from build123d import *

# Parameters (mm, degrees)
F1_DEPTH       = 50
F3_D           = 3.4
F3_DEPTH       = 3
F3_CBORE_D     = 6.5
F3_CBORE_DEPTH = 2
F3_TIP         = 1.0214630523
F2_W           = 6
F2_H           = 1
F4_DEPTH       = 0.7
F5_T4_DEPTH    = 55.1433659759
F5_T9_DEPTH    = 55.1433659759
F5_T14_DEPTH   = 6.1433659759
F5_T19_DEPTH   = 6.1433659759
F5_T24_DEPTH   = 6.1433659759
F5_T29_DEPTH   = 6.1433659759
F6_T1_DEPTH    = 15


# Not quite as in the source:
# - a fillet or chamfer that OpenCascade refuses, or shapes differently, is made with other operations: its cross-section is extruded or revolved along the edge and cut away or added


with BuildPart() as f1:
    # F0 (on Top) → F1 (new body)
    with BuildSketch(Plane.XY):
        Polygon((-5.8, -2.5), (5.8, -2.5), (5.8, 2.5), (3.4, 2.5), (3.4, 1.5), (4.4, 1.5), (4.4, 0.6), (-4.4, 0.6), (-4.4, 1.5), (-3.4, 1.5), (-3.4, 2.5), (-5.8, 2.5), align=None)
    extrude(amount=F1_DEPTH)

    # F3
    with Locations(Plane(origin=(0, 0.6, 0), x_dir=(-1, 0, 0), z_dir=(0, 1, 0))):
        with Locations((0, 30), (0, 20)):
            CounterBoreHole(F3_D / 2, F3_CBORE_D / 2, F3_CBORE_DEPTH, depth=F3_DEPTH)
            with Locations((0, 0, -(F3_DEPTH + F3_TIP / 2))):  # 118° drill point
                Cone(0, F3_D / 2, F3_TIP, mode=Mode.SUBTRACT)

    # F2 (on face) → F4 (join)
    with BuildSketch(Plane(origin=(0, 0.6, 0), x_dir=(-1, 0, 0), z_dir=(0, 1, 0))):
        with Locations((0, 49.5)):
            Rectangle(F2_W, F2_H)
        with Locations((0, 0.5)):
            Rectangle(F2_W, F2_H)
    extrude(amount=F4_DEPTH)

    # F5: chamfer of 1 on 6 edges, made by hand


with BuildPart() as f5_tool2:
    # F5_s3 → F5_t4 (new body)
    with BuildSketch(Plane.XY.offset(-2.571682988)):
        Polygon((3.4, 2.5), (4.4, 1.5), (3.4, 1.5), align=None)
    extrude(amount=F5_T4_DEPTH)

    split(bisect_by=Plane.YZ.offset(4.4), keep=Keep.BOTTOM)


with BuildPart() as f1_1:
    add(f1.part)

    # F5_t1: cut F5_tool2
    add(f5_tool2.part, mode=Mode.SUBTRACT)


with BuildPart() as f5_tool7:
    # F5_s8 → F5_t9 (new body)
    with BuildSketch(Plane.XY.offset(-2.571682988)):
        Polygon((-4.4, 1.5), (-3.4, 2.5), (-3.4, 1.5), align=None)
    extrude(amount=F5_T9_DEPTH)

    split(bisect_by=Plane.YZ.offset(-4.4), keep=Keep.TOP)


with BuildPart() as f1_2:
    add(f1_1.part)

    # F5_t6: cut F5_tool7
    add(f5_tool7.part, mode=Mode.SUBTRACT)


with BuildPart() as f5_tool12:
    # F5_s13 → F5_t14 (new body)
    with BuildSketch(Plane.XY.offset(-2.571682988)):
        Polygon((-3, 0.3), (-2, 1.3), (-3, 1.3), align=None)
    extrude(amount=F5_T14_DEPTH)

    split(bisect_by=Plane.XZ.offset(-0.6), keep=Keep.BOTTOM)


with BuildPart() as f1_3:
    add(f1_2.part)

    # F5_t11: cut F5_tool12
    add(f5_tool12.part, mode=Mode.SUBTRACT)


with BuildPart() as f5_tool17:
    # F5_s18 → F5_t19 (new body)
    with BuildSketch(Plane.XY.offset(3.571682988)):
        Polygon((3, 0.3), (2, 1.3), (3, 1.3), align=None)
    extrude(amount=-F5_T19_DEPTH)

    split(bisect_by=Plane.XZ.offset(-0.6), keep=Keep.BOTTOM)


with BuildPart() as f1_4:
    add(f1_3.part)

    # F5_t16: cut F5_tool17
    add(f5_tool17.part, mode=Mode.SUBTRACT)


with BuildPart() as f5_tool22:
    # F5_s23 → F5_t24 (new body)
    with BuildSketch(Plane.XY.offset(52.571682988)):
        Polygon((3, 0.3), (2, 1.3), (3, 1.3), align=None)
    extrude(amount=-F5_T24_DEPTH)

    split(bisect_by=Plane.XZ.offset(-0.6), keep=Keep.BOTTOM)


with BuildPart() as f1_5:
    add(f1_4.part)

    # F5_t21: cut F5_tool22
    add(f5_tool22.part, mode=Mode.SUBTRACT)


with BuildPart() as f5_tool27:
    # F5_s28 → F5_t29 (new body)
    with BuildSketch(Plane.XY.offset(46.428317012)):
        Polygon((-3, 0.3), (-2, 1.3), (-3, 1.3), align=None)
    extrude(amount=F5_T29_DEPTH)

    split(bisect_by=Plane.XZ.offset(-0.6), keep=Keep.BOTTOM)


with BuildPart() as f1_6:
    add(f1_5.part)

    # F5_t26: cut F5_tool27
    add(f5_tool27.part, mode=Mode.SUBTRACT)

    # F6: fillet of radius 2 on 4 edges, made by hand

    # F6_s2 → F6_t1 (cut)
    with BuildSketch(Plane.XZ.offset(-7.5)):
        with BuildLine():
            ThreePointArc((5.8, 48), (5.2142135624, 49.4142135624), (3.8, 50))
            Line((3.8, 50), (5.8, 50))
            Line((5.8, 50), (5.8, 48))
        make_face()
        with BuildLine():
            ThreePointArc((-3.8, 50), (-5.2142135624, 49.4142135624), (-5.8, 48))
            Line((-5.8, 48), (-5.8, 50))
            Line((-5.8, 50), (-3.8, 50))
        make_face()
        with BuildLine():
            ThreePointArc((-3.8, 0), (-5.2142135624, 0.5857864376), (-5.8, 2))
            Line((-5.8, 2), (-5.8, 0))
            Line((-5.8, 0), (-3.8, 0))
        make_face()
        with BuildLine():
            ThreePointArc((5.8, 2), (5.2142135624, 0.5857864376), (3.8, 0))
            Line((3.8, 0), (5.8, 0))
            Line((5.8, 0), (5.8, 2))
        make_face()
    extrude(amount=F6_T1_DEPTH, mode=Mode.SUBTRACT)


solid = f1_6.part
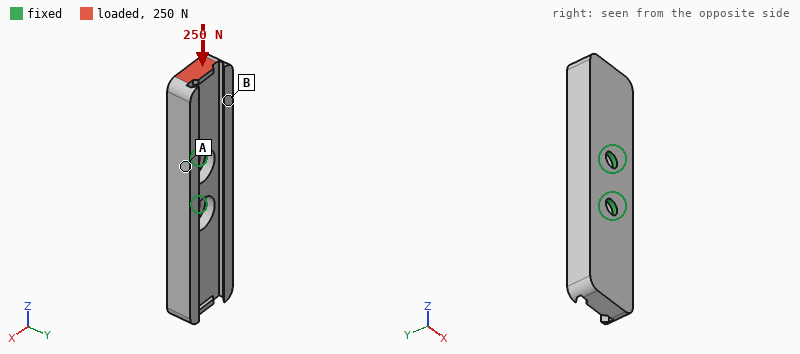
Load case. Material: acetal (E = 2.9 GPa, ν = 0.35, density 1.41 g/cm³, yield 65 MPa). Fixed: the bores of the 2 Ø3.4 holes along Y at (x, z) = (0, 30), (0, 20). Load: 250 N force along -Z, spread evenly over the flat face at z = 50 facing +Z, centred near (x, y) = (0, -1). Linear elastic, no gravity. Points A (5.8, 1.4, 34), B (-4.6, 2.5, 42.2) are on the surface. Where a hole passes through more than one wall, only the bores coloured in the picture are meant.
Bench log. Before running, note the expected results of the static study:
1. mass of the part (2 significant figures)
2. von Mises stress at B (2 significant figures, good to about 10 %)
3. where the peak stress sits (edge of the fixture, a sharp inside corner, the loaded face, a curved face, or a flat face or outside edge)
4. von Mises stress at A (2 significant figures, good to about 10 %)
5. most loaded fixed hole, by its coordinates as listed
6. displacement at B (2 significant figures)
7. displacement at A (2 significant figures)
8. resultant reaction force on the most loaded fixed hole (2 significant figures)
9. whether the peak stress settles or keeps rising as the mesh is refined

2.8 g
3.7 MPa
edge of the fixture
6.9 MPa
(0, 30)
0.097 mm
0.052 mm
180 N
keeps rising
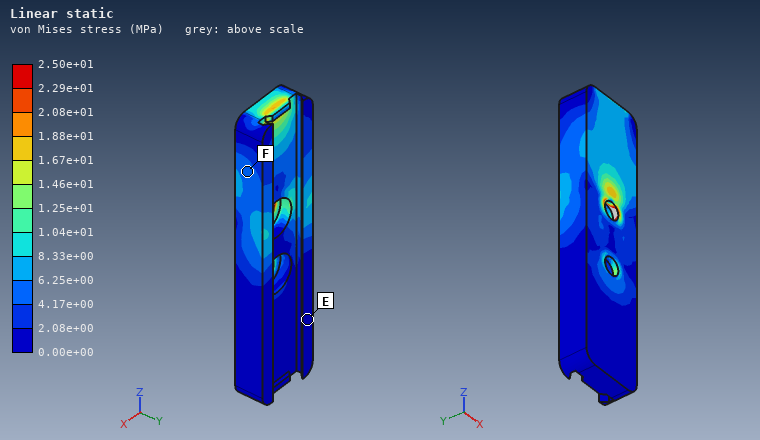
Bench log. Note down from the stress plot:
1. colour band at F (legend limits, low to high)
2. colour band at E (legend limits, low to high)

4.17e+00 to 6.25e+00 MPa
0.00e+00 to 2.08e+00 MPa
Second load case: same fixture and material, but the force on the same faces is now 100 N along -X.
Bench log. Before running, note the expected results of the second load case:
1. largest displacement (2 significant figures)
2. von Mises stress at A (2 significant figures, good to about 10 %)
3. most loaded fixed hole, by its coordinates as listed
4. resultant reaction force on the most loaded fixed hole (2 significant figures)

0.54 mm
17 MPa
(0, 30)
230 N
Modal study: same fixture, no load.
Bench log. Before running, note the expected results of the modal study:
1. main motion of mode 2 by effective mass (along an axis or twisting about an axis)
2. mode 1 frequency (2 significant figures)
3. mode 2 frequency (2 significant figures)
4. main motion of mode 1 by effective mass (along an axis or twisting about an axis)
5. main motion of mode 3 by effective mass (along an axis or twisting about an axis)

along Y
1700 Hz
2000 Hz
twisting about X
along X
